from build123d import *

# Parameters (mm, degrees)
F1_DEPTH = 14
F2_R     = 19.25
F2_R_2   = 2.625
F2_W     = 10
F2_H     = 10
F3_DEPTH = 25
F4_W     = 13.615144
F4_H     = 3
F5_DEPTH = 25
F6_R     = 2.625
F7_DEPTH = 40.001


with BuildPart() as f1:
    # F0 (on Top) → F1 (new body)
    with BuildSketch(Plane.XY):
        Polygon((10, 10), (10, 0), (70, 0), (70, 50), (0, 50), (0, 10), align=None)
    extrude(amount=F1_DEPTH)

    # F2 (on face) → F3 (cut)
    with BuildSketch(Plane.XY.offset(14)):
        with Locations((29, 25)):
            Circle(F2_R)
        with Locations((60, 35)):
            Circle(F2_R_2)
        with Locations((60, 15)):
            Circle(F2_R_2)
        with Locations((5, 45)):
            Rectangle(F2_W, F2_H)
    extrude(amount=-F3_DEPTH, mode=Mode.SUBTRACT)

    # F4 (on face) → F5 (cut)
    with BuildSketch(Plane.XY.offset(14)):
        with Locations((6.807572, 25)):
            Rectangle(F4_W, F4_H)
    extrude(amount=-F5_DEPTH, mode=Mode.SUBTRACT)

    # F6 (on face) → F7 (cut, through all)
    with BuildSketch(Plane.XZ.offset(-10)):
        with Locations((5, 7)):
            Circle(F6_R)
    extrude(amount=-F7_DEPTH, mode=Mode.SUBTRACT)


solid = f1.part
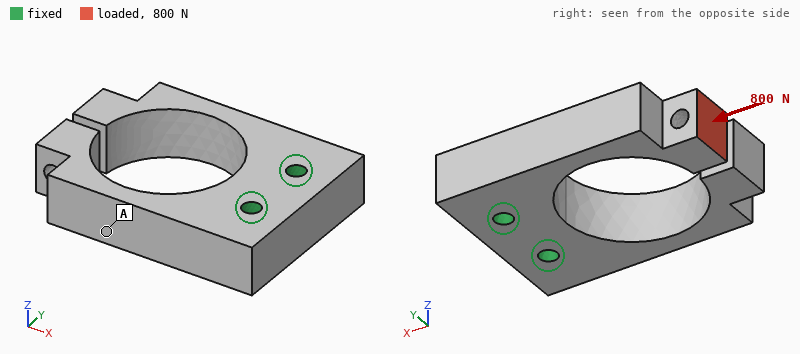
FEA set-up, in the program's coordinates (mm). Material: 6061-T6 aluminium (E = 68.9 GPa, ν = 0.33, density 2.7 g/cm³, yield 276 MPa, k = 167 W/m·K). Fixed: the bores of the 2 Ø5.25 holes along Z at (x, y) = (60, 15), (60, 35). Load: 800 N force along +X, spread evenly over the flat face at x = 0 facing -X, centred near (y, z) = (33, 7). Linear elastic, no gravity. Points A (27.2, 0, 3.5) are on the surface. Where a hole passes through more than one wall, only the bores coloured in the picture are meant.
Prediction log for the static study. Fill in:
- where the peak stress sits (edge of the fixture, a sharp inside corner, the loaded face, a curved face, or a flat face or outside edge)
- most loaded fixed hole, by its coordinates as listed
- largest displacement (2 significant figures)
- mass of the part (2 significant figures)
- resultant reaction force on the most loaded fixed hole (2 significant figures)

a curved face
(60, 35)
0.48 mm
76 g
720 N
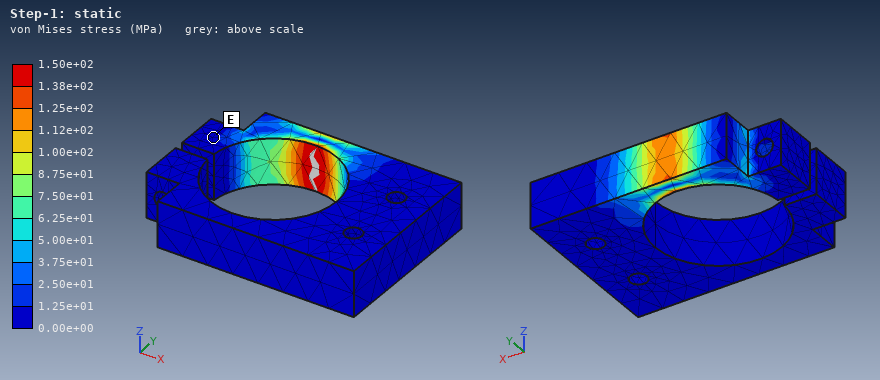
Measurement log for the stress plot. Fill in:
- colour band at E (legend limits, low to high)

0.00e+00 to 1.25e+01 MPa
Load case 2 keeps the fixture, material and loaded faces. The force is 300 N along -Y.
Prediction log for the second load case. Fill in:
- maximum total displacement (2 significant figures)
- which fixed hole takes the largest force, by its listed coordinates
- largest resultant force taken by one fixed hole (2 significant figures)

0.43 mm
(60, 15)
720 N
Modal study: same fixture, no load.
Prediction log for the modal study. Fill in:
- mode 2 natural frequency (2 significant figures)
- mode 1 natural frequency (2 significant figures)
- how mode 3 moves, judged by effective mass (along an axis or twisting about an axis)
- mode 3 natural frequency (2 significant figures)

1900 Hz
1900 Hz
along Z
2600 Hz
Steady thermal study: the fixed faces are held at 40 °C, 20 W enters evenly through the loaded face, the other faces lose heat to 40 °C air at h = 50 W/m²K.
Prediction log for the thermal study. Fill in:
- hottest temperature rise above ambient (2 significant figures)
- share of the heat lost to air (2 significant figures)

57 K
23 %
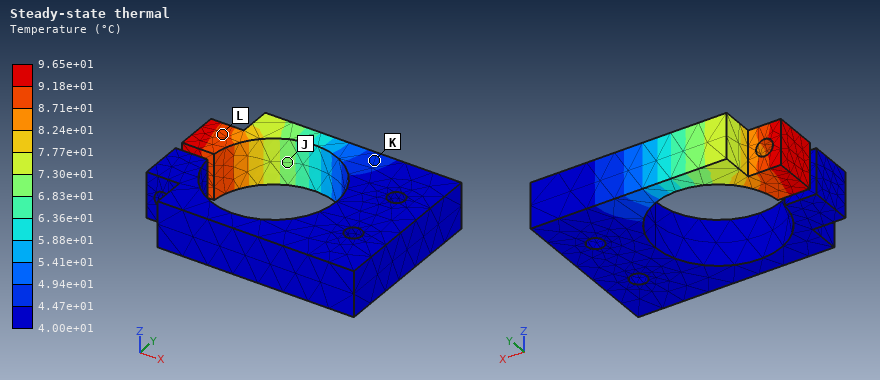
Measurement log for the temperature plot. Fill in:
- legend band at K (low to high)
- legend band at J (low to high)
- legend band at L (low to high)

4.47e+01 to 4.94e+01 °C
6.83e+01 to 7.30e+01 °C
8.71e+01 to 9.18e+01 °C
